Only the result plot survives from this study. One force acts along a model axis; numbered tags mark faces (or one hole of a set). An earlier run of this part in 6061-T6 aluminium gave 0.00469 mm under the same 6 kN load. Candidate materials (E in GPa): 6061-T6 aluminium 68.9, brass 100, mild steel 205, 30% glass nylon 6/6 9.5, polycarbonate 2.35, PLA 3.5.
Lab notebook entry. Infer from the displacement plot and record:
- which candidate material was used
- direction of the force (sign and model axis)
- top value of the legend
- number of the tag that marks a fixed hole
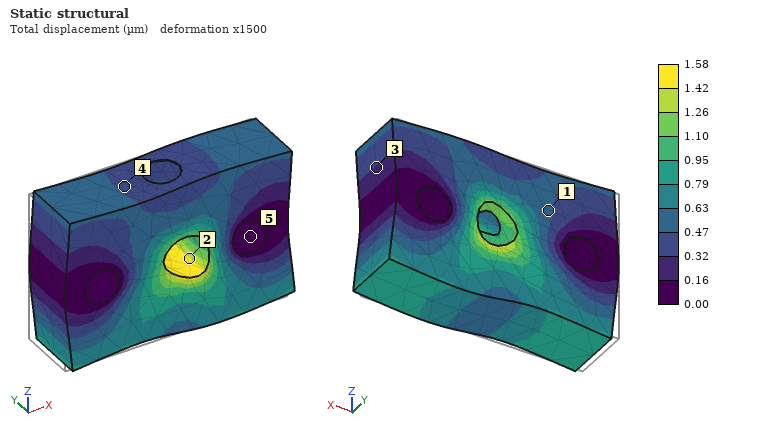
mild steel
+X
1.58 µm
5
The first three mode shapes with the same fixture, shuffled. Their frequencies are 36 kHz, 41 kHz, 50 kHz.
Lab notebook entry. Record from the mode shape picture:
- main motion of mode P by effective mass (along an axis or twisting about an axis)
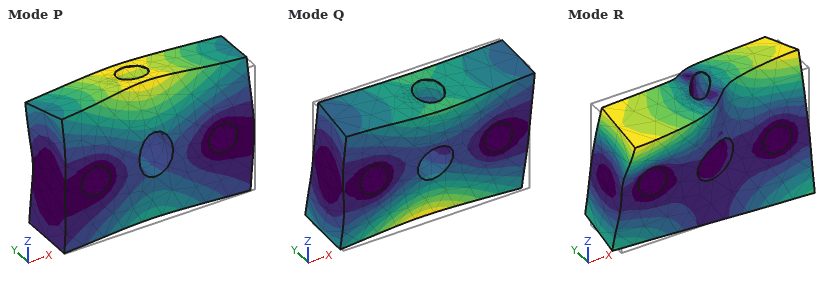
along Y
